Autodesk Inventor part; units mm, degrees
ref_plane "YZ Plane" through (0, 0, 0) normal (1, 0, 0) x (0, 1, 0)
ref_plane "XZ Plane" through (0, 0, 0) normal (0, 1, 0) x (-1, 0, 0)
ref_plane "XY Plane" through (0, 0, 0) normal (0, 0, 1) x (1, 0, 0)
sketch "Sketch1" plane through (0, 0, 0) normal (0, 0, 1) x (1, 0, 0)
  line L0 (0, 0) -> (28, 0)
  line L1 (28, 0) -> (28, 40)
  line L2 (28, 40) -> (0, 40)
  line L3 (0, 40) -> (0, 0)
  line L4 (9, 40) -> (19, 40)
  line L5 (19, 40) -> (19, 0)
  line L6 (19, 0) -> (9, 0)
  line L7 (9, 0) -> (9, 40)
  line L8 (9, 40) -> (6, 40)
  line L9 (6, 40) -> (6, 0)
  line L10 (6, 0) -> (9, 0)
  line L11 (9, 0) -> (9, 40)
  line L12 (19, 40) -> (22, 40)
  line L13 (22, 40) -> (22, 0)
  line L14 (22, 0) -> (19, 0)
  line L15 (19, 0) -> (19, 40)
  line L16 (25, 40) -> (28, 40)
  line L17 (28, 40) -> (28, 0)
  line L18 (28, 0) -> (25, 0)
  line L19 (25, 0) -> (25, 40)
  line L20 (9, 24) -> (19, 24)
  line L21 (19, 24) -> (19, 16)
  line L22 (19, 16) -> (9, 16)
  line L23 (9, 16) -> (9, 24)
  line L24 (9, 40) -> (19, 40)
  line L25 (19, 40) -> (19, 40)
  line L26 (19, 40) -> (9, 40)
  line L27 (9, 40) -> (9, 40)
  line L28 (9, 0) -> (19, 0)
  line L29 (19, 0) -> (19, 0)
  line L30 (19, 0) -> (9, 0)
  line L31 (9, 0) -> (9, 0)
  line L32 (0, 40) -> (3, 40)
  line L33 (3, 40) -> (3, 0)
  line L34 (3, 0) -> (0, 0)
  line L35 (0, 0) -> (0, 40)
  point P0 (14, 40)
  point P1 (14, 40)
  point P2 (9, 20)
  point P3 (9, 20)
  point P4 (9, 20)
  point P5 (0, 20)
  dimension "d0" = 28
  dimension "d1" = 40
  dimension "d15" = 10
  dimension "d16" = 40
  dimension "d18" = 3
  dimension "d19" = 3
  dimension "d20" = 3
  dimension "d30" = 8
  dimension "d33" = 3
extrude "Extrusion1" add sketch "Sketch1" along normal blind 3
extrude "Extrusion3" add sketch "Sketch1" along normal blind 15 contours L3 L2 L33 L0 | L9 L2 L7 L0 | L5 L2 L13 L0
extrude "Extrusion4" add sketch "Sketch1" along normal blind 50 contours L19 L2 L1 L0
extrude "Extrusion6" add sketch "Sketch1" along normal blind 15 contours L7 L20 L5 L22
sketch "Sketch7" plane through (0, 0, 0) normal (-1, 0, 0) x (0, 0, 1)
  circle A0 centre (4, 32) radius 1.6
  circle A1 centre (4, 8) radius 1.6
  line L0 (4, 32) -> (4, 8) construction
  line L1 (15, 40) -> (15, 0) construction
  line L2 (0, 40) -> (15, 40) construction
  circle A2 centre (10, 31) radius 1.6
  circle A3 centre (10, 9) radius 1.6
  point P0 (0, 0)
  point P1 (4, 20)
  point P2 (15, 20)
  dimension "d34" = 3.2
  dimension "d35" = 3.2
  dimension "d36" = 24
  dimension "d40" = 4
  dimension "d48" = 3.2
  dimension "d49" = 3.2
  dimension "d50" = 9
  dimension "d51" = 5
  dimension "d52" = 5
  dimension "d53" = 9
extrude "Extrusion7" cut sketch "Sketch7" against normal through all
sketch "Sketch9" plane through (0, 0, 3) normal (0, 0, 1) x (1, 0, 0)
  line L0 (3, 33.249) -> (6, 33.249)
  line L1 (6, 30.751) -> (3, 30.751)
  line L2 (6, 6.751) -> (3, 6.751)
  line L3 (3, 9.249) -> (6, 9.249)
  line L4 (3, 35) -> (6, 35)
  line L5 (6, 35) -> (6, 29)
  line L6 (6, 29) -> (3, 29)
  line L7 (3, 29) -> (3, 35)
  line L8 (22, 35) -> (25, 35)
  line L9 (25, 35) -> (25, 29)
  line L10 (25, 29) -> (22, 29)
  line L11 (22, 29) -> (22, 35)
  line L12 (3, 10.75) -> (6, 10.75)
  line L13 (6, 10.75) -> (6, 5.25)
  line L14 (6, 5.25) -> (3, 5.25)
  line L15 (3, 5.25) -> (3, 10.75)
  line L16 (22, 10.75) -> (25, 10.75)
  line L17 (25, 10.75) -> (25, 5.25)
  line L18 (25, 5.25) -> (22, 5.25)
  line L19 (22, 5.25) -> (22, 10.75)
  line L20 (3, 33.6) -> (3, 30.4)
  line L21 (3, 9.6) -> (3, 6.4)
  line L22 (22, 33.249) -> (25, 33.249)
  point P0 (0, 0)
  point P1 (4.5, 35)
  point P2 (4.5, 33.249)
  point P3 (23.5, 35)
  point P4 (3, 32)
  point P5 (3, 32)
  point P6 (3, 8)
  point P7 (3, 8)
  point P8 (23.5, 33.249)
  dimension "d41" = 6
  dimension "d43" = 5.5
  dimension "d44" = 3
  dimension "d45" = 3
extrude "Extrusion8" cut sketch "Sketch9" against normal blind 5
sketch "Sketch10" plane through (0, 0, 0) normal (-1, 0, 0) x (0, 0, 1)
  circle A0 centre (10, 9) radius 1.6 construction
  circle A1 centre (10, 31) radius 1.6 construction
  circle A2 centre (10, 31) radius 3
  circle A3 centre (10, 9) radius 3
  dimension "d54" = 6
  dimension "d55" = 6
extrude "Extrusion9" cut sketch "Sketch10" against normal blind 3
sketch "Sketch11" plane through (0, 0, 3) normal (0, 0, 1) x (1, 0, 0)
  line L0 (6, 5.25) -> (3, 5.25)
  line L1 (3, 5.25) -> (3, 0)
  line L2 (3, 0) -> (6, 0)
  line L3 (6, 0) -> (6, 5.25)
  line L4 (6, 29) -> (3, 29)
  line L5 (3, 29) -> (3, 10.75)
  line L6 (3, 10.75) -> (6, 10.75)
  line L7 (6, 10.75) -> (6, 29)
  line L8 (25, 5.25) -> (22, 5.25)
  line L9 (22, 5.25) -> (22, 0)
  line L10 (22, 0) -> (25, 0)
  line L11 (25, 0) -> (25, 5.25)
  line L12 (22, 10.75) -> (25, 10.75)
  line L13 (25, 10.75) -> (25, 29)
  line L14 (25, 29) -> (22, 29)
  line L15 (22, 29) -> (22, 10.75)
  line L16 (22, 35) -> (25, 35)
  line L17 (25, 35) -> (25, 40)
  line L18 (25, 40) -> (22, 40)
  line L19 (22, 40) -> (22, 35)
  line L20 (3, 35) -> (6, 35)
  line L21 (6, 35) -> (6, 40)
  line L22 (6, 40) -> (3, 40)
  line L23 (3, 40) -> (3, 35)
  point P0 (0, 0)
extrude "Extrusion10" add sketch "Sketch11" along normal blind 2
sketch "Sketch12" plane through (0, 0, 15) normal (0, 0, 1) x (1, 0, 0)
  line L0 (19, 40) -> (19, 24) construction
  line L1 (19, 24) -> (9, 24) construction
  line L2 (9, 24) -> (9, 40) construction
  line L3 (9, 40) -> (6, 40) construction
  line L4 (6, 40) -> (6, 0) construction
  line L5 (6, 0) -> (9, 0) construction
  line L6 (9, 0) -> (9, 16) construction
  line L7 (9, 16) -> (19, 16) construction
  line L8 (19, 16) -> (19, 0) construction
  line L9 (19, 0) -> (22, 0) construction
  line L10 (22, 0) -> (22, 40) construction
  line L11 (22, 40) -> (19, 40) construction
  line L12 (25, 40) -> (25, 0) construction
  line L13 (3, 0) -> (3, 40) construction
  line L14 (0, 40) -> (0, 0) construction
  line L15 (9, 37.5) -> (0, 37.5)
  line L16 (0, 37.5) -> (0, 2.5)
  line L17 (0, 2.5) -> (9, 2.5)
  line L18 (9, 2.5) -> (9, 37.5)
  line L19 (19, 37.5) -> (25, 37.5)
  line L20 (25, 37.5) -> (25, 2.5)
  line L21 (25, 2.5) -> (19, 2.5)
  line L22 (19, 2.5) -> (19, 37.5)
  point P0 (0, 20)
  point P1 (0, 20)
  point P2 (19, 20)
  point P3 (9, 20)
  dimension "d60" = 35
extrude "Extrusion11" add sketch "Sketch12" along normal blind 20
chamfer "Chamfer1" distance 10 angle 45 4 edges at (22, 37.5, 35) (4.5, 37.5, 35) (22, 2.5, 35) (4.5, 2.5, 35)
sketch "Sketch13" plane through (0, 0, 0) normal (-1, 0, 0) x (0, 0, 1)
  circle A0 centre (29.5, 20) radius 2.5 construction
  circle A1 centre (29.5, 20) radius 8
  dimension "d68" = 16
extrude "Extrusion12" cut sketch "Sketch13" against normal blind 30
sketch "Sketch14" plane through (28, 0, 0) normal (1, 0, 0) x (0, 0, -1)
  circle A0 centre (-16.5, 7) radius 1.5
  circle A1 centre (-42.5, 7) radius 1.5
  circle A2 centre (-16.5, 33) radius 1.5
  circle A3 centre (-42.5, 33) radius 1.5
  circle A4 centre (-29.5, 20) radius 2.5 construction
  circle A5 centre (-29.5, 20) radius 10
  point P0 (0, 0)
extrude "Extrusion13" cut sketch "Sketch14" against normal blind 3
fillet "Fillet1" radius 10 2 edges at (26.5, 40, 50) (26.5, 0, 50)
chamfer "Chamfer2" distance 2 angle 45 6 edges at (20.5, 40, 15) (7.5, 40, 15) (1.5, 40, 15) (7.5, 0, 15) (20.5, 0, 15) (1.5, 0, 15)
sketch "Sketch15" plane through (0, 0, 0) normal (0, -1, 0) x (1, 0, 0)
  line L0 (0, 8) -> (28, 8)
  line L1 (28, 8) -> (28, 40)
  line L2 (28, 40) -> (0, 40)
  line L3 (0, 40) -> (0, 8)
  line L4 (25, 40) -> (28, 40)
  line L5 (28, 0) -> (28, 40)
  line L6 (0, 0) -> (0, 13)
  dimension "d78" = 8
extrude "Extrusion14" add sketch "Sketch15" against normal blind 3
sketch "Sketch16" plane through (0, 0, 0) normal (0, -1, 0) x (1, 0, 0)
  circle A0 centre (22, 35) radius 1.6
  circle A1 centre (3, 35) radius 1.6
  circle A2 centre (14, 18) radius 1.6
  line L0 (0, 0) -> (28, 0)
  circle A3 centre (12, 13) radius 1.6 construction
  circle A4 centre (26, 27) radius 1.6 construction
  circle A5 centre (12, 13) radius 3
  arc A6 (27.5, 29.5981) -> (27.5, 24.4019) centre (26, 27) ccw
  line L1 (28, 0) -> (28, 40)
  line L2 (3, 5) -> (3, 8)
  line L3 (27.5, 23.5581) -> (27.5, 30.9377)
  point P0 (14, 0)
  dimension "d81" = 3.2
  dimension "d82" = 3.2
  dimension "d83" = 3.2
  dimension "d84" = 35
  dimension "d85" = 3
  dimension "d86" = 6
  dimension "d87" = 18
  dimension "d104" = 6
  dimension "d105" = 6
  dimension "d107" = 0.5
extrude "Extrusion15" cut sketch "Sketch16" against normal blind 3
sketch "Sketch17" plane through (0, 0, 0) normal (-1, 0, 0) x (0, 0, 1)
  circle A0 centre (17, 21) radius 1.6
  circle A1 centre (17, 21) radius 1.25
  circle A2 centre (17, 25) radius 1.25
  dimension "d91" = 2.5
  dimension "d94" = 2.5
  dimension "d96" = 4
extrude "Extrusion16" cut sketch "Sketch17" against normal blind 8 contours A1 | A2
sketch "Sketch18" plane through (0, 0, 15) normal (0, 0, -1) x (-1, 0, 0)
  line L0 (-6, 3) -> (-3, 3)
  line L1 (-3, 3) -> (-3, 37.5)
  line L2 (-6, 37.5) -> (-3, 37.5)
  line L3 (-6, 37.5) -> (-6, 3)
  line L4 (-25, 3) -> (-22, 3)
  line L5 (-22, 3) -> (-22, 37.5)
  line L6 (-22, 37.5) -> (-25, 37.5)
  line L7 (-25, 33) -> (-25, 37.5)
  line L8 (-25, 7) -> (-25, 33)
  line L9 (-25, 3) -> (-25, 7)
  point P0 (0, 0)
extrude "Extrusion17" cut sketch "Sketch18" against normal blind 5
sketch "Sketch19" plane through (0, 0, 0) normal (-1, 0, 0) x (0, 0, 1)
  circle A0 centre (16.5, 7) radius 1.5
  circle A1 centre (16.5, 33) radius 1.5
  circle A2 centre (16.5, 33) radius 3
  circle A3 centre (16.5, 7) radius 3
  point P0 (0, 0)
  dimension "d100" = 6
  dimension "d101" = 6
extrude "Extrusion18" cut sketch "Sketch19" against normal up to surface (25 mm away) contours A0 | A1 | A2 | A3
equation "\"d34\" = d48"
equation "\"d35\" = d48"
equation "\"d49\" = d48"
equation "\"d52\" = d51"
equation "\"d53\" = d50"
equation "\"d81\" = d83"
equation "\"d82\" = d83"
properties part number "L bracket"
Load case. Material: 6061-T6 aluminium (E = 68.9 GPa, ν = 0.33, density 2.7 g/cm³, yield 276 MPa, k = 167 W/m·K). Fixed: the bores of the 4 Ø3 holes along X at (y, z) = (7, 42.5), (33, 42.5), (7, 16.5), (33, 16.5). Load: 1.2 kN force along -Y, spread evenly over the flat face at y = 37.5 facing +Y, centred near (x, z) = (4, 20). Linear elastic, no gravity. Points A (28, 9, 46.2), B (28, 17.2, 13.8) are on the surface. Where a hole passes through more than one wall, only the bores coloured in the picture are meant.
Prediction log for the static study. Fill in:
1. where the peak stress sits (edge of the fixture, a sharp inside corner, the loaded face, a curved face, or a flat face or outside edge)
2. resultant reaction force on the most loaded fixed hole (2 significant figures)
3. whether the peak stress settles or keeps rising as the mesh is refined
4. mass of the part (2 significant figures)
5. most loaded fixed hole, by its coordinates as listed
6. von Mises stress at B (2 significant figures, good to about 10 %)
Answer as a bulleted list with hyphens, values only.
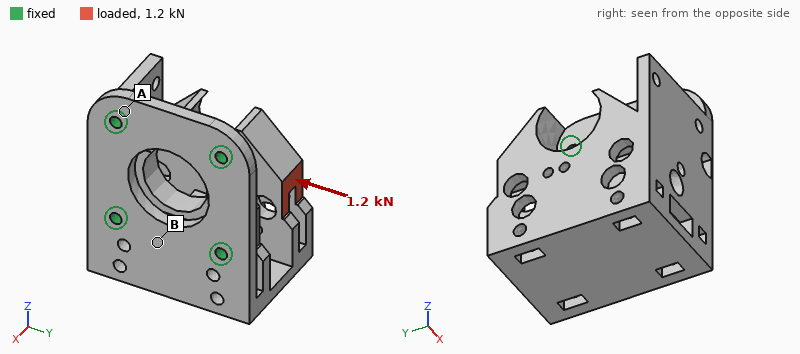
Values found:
- edge of the fixture
- 1.1 kN
- keeps rising
- 52 g
- (33, 16.5)
- 28 MPa
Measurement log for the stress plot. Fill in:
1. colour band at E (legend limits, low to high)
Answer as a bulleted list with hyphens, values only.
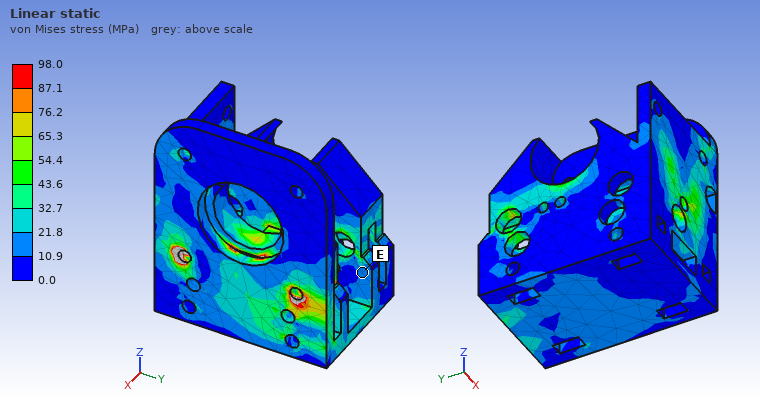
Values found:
- 10.9 to 21.8 MPa
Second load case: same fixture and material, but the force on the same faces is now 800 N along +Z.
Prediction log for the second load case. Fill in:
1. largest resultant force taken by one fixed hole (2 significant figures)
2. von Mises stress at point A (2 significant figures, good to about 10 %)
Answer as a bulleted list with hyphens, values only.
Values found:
- 630 N
- 9.9 MPa
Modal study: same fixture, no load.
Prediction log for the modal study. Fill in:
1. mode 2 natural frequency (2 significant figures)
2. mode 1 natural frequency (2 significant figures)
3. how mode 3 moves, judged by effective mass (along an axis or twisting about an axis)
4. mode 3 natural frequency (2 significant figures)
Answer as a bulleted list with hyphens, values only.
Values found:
- 4100 Hz
- 3800 Hz
- along X
- 6600 Hz
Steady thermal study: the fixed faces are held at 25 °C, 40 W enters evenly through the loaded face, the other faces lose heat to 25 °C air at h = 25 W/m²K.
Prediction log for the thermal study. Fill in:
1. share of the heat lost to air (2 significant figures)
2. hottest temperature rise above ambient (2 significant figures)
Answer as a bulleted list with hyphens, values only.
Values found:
- 16 %
- 80 K
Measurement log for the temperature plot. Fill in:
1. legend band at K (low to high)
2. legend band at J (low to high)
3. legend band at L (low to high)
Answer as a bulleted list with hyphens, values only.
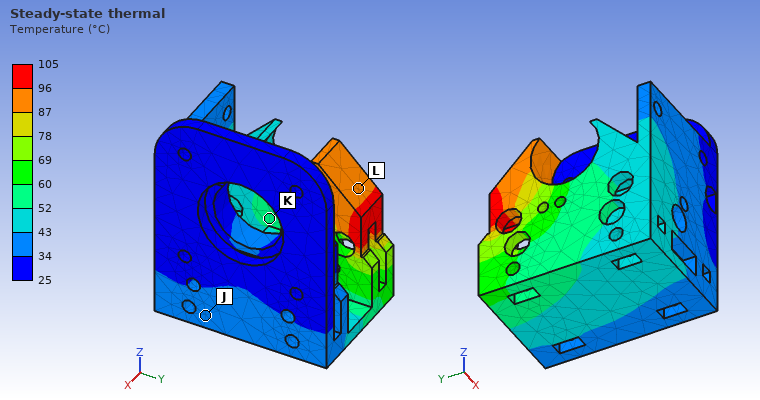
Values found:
- 52 to 60 °C
- 34 to 43 °C
- 87 to 96 °C
